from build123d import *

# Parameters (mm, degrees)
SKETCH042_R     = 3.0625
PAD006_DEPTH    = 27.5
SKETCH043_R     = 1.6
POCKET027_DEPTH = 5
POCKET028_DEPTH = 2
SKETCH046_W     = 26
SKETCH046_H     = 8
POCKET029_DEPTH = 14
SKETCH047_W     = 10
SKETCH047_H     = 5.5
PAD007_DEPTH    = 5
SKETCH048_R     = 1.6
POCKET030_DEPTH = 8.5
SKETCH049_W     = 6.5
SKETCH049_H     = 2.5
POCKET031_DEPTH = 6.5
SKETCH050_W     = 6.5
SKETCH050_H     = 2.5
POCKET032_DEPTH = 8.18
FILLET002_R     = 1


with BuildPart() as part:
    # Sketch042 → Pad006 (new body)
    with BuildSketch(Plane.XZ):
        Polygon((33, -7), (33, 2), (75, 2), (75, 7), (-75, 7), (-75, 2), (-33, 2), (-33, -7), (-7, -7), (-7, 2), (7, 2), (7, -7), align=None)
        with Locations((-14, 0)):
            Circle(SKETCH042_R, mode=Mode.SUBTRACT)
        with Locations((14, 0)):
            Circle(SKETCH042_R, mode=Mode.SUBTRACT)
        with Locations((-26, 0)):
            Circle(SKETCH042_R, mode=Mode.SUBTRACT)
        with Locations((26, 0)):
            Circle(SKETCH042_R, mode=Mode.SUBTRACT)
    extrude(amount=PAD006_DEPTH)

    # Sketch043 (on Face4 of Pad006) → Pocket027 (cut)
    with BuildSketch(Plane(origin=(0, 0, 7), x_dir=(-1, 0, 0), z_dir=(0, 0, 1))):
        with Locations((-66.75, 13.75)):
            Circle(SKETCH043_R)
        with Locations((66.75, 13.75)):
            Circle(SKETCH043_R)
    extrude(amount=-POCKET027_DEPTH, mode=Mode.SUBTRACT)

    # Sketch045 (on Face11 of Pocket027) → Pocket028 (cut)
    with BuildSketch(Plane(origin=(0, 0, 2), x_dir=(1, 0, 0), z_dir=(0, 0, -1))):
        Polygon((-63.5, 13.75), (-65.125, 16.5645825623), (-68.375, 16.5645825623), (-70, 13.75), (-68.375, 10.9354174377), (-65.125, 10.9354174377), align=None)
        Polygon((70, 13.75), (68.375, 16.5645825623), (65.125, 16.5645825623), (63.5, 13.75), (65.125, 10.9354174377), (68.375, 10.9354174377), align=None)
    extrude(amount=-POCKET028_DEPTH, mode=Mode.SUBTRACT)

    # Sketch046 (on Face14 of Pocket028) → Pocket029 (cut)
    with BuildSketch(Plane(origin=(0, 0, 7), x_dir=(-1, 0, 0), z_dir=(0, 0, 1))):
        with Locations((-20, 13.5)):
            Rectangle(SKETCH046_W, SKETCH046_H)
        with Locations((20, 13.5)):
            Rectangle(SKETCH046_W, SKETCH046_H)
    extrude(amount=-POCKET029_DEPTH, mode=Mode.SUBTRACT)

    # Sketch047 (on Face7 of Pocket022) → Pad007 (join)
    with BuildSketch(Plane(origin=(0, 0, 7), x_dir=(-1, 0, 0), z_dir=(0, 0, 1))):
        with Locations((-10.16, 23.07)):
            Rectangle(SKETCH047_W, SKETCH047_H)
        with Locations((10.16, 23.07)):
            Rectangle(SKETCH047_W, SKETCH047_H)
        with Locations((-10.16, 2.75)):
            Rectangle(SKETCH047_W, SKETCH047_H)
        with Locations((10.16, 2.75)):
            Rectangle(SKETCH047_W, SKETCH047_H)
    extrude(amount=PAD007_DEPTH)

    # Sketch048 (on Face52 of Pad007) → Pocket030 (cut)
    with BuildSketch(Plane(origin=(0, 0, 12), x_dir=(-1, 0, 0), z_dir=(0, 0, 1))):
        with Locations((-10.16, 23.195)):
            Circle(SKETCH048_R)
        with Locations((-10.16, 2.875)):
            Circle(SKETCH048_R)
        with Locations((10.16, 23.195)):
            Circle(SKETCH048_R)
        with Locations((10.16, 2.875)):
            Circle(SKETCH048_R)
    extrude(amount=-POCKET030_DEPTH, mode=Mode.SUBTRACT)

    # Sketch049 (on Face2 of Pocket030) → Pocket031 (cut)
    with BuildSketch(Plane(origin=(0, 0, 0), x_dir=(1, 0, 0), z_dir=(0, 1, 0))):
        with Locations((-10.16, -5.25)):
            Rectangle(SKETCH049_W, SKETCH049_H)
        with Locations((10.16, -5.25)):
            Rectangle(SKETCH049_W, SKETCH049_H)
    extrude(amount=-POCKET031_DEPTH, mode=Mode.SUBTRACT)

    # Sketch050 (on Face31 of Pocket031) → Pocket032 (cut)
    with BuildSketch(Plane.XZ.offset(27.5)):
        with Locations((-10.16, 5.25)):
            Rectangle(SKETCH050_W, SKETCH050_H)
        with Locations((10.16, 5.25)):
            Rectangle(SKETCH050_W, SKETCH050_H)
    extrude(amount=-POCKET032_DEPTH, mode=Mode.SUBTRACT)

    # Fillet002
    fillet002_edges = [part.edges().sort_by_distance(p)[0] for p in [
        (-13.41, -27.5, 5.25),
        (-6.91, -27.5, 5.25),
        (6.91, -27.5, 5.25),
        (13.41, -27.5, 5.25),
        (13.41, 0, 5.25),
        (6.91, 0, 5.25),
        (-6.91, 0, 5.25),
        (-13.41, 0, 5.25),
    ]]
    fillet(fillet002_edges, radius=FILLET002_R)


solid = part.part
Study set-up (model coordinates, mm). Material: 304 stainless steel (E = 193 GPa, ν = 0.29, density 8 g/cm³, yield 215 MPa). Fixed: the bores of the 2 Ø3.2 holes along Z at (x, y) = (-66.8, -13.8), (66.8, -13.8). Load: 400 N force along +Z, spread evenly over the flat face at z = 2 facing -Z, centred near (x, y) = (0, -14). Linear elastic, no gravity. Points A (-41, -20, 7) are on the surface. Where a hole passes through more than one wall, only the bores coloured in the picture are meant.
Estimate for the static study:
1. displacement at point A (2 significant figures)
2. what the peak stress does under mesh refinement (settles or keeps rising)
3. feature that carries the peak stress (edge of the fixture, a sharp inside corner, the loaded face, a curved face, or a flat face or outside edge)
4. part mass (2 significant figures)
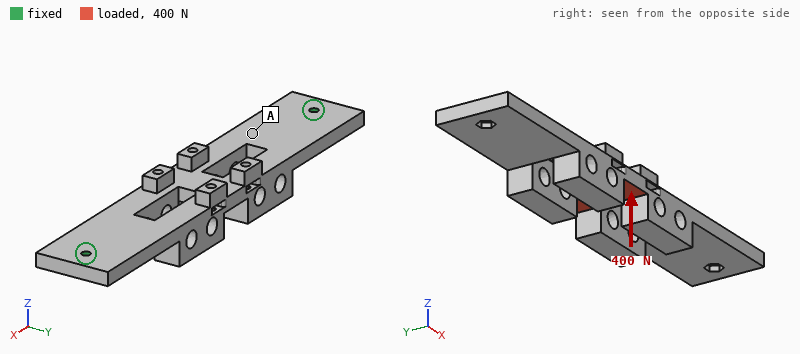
0.044 mm
keeps rising
edge of the fixture
210 g
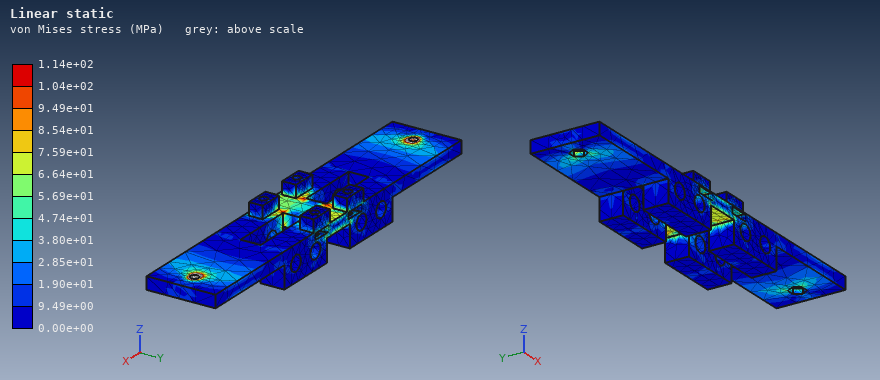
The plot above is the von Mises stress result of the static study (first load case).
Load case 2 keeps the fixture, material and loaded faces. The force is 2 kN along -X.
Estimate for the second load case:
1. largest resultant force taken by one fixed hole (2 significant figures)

1.0 kN
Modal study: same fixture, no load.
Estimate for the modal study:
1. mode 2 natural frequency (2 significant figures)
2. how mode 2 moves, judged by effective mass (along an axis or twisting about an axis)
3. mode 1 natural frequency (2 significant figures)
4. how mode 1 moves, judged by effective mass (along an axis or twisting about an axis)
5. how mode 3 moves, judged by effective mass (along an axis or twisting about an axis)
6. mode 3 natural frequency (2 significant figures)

2000 Hz
along Y
1000 Hz
along Z
along Y
2800 Hz
